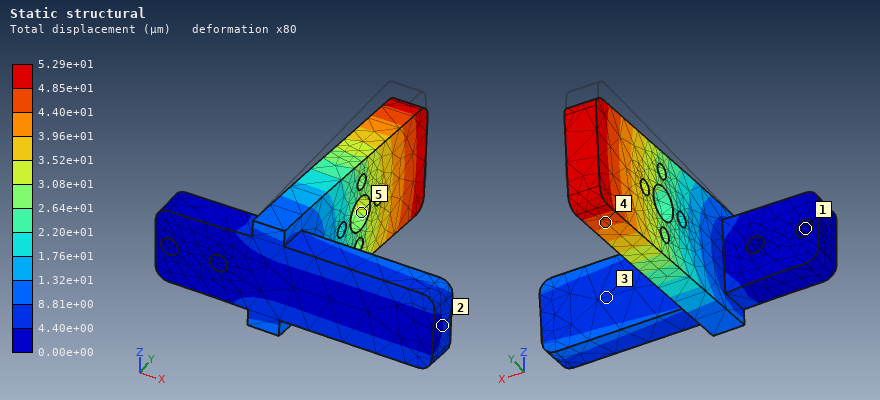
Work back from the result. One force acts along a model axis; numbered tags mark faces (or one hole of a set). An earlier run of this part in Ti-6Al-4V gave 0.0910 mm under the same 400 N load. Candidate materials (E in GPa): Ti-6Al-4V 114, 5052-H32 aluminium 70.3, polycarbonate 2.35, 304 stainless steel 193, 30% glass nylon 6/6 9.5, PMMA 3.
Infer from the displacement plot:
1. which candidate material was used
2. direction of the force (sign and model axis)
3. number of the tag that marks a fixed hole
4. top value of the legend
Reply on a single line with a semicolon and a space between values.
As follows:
304 stainless steel; -Z; 1; 5.29e+01 µm
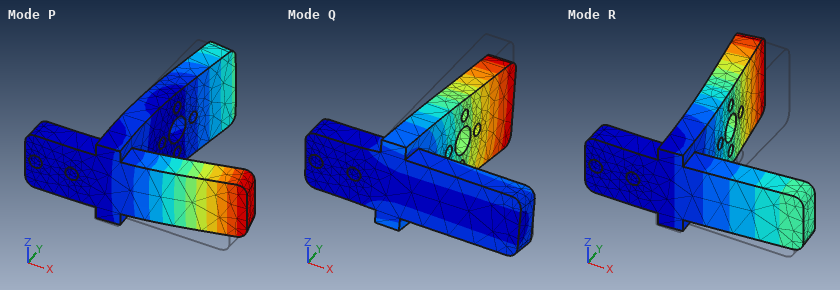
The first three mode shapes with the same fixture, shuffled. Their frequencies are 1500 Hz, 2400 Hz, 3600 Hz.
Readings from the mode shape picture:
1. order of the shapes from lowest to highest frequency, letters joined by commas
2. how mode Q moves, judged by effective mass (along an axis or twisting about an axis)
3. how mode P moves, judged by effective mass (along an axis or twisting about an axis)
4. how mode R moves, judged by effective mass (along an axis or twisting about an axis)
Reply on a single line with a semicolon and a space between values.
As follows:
R, Q, P; along Z; along Y; along X
